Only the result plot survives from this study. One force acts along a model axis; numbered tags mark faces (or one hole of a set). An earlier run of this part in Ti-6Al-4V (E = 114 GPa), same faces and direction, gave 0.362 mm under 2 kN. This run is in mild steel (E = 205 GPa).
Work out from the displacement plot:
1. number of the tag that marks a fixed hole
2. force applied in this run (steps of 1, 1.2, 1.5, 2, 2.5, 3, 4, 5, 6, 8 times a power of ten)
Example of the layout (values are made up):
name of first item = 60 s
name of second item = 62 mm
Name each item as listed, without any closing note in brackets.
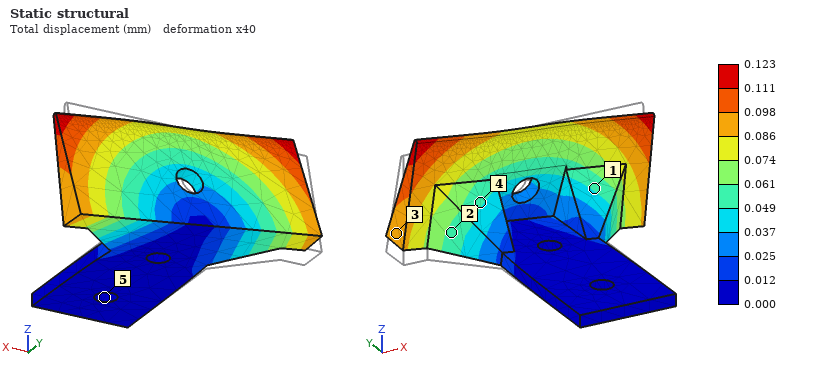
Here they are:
number of the tag that marks a fixed hole = 5
force applied in this run = 1.2 kN
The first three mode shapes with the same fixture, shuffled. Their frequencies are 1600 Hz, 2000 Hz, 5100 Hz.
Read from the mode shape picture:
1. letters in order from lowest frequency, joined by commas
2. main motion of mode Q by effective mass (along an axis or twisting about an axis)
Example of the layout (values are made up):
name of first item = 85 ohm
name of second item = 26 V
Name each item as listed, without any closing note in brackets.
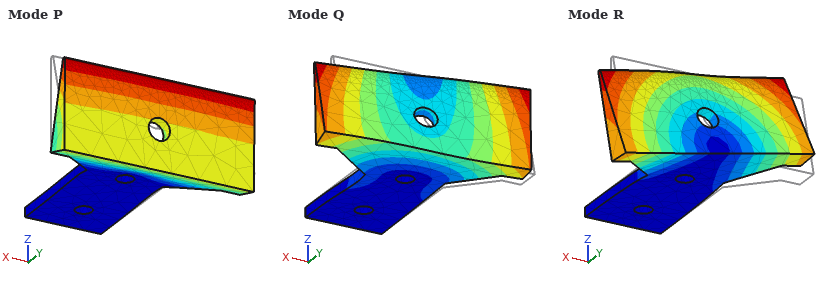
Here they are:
letters in order from lowest frequency, joined by commas = R, P, Q
main motion of mode Q by effective mass = along X
